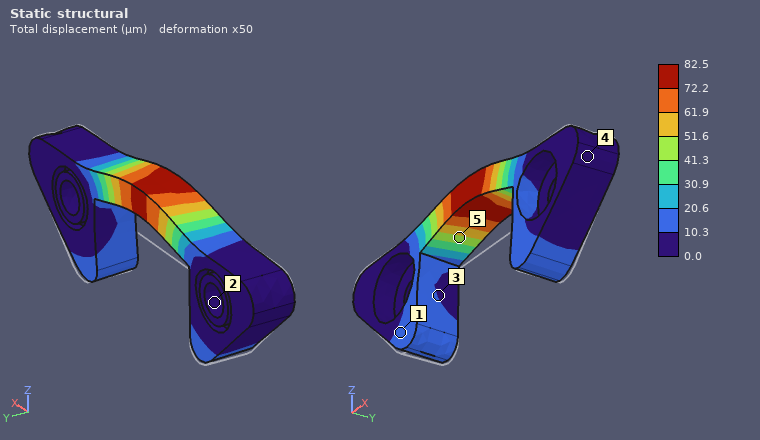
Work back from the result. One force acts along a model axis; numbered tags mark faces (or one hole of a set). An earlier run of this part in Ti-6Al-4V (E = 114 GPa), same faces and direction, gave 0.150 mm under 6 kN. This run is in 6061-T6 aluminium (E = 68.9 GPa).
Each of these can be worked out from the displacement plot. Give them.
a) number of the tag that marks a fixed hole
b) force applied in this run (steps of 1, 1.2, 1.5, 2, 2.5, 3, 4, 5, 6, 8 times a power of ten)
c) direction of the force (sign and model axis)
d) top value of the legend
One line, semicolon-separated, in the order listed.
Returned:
2; 2 kN; +Z; 82.5 µm
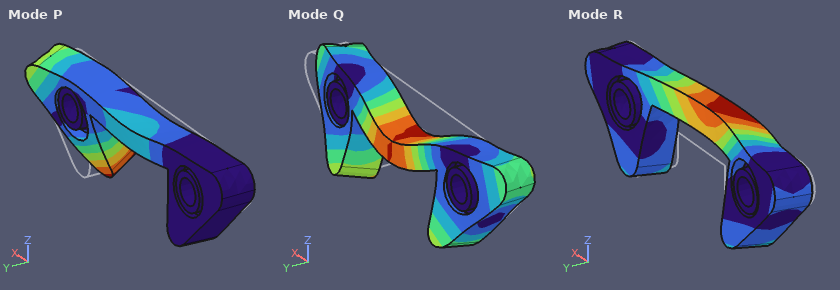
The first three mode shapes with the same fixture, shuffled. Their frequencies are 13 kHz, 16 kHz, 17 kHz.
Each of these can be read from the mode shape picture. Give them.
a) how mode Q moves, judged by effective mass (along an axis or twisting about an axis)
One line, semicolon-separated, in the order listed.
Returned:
along Z
